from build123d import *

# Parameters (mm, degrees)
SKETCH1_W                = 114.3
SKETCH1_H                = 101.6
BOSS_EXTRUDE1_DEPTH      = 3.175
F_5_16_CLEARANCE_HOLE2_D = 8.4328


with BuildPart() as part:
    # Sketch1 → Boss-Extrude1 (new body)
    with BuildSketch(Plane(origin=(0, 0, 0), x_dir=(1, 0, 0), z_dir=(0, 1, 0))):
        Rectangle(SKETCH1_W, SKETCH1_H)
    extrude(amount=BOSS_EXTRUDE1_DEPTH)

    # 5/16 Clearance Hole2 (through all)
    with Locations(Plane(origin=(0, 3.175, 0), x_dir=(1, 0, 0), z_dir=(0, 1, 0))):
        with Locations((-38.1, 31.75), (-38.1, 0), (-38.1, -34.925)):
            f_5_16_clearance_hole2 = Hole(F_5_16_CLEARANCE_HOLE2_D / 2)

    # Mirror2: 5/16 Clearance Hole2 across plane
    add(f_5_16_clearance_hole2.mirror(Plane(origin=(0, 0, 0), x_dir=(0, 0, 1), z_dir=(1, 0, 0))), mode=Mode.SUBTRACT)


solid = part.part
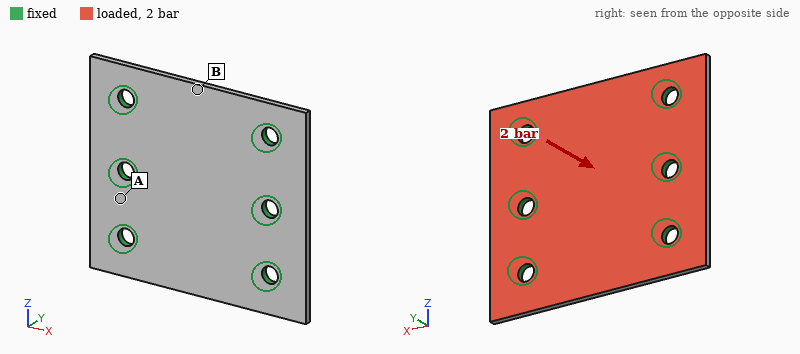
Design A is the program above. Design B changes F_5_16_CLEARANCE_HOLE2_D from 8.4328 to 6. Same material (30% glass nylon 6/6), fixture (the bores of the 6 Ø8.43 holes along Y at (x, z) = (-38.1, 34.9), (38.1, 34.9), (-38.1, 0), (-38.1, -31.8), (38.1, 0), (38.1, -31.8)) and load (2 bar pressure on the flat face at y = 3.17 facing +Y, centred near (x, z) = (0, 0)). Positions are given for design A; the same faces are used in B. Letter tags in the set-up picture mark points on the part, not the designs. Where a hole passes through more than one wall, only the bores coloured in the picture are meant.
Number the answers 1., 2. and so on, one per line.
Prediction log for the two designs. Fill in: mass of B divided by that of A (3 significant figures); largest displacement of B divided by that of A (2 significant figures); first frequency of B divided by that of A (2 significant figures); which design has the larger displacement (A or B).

1. 1.01
2. 1.2
3. 0.92
4. B
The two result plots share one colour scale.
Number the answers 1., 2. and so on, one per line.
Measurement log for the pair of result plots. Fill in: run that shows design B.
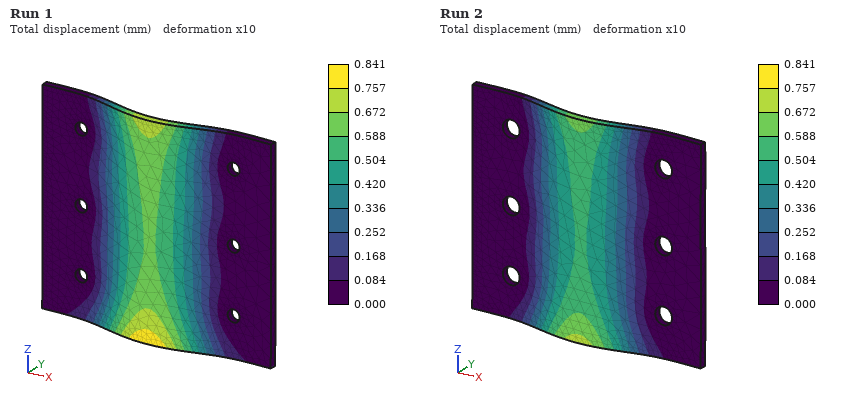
1. Run 1
